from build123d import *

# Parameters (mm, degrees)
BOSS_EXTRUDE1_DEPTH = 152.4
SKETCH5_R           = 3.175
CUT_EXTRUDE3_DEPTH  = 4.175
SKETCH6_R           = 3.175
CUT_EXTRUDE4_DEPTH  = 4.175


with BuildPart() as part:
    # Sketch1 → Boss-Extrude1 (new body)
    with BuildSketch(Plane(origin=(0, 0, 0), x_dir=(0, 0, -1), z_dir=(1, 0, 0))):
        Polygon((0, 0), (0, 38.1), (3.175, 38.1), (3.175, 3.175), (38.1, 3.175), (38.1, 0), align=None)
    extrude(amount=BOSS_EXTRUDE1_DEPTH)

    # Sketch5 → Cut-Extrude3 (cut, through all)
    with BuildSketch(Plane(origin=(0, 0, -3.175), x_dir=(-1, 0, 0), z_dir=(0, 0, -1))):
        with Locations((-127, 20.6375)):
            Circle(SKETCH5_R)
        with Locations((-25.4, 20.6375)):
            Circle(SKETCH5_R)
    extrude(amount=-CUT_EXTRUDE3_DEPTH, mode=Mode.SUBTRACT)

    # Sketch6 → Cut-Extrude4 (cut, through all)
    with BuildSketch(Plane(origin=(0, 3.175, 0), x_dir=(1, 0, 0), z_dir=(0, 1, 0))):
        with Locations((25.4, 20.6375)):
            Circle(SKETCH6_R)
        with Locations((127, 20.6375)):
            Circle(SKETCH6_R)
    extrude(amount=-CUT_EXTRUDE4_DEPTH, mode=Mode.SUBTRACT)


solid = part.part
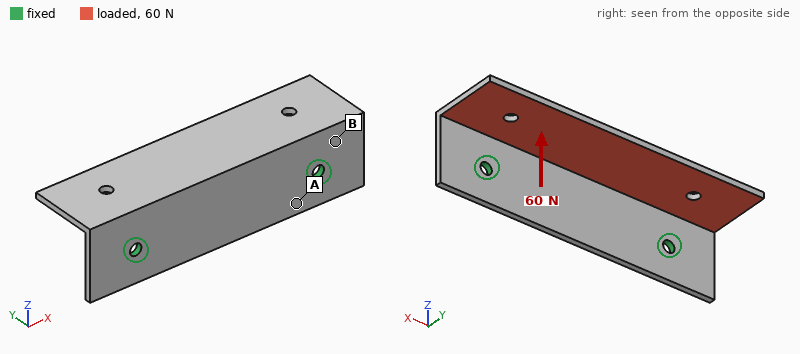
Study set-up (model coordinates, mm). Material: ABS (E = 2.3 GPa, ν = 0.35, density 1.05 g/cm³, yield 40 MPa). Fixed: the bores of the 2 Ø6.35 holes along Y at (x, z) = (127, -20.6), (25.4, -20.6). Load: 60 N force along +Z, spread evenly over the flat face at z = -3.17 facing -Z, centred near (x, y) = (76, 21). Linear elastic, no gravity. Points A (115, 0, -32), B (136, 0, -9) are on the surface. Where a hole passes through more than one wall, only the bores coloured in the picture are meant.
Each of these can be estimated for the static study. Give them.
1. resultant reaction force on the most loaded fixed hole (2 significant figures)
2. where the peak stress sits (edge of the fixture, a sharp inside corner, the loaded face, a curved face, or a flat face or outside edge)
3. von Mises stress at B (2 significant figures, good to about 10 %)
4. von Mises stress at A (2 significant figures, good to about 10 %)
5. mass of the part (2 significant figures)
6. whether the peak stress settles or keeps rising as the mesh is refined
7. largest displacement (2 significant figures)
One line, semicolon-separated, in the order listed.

30 N; edge of the fixture; 4.8 MPa; 1.5 MPa; 37 g; keeps rising; 1.5 mm
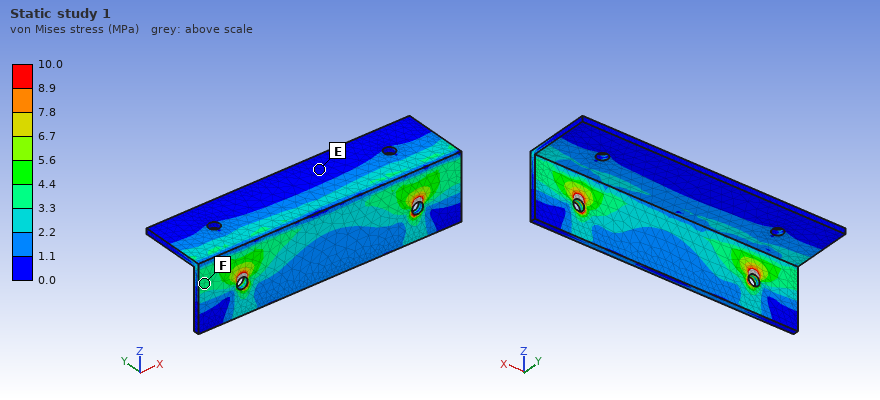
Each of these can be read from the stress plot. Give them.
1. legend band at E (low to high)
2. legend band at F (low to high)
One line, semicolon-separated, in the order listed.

0.0 to 1.1 MPa; 3.3 to 4.4 MPa
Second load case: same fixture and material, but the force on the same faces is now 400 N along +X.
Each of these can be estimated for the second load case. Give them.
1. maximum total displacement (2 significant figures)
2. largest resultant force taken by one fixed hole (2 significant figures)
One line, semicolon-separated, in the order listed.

1.7 mm; 220 N
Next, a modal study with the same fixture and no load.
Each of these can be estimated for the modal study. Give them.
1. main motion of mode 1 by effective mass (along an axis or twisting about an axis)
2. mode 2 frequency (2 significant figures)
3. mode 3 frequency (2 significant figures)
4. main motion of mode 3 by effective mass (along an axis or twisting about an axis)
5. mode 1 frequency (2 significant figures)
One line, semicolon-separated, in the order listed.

along Z; 400 Hz; 600 Hz; along Y; 280 Hz
